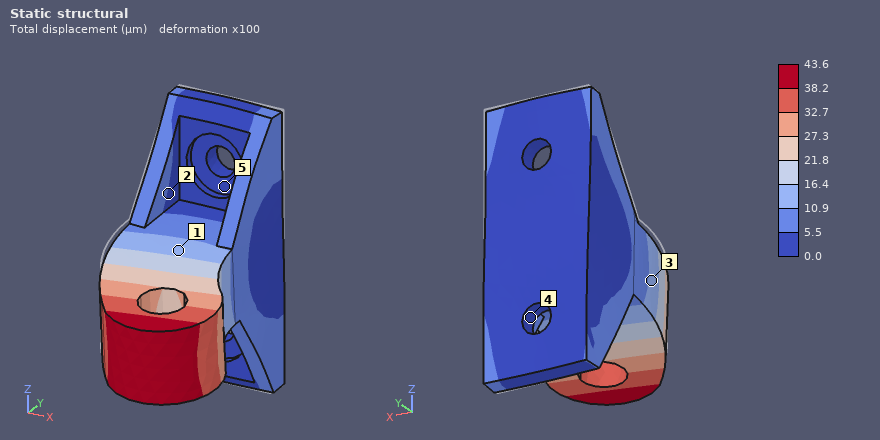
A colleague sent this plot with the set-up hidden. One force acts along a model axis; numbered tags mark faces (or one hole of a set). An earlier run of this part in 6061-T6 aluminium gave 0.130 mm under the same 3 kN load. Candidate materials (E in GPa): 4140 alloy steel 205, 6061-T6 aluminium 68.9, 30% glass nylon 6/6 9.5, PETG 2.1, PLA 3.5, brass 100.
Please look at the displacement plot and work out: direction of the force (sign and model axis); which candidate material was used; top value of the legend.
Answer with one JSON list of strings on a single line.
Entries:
["-Z", "4140 alloy steel", "43.6 µm"]
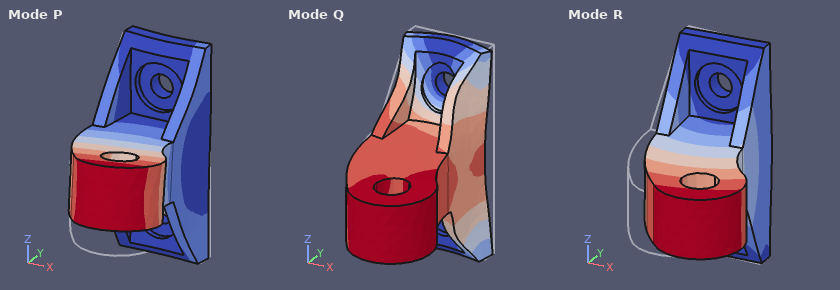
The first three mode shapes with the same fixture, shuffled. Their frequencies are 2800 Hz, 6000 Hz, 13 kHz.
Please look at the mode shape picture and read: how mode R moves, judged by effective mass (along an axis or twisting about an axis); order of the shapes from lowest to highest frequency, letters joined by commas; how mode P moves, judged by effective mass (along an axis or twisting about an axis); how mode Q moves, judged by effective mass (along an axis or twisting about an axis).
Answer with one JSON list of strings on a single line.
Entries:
["along X", "R, P, Q", "along Z", "along Y"]
